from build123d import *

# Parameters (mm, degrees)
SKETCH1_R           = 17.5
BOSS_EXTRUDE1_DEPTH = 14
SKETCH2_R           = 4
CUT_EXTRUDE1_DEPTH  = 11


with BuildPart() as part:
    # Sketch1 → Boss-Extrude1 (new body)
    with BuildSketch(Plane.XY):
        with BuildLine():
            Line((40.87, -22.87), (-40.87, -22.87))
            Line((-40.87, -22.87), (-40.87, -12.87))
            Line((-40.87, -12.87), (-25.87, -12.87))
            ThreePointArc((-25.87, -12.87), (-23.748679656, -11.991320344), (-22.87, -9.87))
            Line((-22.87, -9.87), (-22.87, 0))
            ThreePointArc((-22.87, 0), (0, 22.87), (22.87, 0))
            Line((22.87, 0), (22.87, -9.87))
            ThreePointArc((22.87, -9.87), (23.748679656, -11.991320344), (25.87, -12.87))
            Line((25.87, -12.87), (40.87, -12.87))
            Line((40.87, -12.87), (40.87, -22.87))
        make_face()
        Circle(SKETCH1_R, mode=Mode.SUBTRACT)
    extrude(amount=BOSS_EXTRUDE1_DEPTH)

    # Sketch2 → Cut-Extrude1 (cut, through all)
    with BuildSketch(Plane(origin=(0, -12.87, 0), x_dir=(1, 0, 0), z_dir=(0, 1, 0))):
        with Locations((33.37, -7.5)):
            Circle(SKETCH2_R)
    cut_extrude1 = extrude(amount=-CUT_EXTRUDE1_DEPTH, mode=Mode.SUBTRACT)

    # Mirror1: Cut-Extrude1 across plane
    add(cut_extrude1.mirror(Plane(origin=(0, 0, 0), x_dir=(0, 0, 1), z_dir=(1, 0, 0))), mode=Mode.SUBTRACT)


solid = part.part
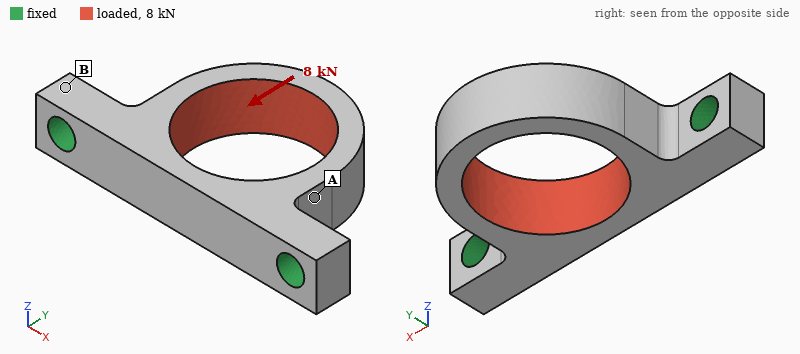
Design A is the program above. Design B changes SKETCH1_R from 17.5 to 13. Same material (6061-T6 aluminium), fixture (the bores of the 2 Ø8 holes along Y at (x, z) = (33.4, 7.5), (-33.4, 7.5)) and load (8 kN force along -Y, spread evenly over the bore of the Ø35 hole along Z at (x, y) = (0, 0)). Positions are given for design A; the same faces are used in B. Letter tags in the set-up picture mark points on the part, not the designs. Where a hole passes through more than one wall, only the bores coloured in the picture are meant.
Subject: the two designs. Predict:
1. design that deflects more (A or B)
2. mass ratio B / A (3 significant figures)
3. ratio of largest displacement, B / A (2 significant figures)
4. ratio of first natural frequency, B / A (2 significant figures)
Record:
A
1.36
0.66
0.89
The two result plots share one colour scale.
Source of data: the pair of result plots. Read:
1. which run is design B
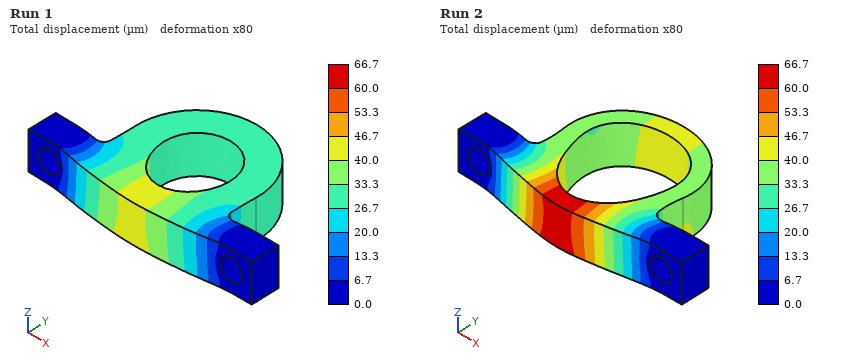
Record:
Run 1
